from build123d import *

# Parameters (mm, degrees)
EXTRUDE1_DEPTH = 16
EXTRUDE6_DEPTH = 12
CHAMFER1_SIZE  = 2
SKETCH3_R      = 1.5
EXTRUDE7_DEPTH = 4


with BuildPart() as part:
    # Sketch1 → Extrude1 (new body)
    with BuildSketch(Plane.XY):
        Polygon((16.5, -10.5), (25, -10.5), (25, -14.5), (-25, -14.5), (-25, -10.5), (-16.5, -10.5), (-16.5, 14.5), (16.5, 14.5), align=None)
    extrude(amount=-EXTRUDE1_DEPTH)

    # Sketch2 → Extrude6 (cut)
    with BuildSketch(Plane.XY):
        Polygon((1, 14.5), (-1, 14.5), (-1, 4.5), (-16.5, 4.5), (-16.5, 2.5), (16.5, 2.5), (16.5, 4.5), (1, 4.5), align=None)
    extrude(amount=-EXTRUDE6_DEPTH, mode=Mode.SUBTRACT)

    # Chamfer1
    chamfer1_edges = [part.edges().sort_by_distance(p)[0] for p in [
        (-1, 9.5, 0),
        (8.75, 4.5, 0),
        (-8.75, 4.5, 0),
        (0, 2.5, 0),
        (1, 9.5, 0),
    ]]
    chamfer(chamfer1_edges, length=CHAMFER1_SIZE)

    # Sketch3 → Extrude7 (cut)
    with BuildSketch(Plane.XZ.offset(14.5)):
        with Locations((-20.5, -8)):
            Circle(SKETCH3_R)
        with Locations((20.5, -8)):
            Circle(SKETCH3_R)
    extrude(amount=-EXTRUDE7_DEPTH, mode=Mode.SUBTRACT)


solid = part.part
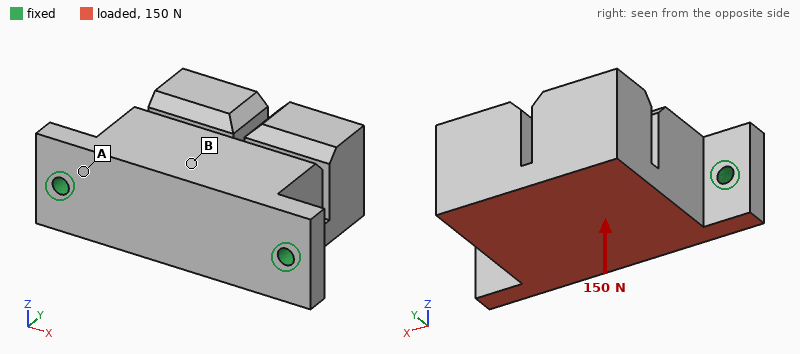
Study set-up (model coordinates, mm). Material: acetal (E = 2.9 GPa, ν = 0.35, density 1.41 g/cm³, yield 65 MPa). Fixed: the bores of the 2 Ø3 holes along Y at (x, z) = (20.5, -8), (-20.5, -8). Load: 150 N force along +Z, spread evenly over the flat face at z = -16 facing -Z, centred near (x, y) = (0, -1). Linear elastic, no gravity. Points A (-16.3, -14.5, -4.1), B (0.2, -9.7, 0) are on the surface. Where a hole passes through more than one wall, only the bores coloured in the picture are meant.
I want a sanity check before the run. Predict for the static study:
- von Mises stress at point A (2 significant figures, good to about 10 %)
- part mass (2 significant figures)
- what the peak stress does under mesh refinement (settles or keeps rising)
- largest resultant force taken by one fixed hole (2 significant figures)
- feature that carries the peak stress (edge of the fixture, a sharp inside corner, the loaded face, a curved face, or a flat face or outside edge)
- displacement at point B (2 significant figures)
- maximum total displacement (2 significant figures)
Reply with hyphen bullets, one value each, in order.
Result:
- 5.7 MPa
- 21 g
- keeps rising
- 75 N
- edge of the fixture
- 0.12 mm
- 0.46 mm
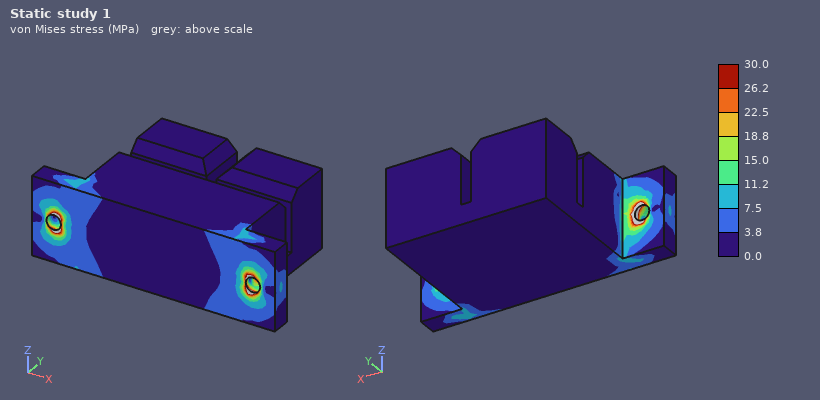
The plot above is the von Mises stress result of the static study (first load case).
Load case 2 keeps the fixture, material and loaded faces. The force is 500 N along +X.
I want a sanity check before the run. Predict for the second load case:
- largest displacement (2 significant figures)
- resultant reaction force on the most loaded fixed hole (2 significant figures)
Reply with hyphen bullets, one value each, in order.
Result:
- 0.11 mm
- 310 N
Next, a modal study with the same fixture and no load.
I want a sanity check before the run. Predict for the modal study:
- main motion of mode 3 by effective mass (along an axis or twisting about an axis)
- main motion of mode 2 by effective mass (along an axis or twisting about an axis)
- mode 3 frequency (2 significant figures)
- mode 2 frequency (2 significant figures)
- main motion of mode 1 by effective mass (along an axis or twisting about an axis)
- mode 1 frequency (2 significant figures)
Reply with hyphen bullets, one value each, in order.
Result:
- along X
- along Y
- 2600 Hz
- 2200 Hz
- along Z
- 770 Hz
